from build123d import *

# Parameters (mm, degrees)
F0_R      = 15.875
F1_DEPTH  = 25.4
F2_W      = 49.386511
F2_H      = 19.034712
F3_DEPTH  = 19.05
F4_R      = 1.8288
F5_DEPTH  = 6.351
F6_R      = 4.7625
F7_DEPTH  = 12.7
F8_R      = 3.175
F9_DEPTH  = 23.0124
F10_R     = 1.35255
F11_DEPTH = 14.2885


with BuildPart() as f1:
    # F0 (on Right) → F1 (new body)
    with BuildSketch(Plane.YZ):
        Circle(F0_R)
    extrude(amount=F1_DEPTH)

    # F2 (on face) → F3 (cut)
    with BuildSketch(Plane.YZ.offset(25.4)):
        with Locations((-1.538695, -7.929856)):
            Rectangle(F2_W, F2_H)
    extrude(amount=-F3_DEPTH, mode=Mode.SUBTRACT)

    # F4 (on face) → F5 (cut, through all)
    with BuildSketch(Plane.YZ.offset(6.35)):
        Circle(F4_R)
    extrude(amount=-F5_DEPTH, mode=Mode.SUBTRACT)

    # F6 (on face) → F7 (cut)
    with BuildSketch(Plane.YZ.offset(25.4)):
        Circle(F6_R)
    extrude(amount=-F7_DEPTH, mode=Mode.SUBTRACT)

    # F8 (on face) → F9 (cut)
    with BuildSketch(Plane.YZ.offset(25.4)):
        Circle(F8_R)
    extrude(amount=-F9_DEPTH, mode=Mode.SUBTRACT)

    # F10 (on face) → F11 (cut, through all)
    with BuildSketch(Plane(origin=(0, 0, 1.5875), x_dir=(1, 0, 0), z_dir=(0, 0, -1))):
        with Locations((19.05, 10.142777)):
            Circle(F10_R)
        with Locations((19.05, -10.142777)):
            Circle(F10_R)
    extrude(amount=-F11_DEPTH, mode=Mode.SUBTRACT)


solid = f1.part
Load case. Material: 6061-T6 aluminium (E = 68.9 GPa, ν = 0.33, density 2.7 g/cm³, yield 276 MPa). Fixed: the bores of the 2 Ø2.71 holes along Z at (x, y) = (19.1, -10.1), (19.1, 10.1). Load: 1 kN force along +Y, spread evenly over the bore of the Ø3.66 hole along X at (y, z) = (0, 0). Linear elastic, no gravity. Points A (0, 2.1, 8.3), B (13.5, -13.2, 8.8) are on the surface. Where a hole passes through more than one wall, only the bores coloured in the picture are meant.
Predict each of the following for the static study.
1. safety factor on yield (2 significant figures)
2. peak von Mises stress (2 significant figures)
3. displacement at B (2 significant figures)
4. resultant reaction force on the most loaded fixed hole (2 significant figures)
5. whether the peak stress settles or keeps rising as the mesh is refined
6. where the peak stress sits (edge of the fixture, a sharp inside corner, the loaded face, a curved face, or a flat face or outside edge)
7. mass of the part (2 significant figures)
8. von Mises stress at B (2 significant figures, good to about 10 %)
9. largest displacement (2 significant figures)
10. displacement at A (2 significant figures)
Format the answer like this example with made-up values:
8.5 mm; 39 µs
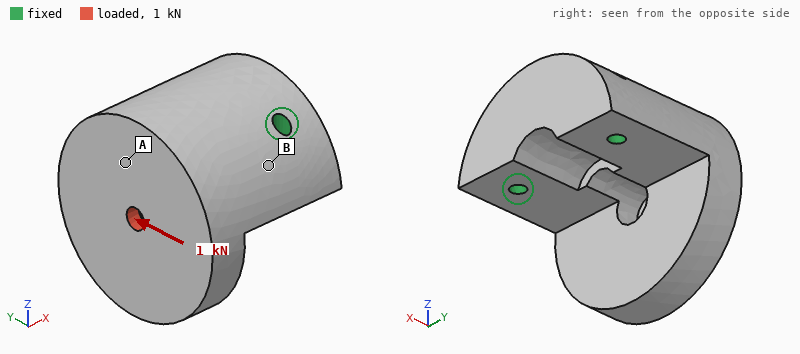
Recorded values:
4.1; 67 MPa; 2.5 µm; 1.0 kN; settles; the loaded face; 30 g; 15 MPa; 13 µm; 4.0 µm
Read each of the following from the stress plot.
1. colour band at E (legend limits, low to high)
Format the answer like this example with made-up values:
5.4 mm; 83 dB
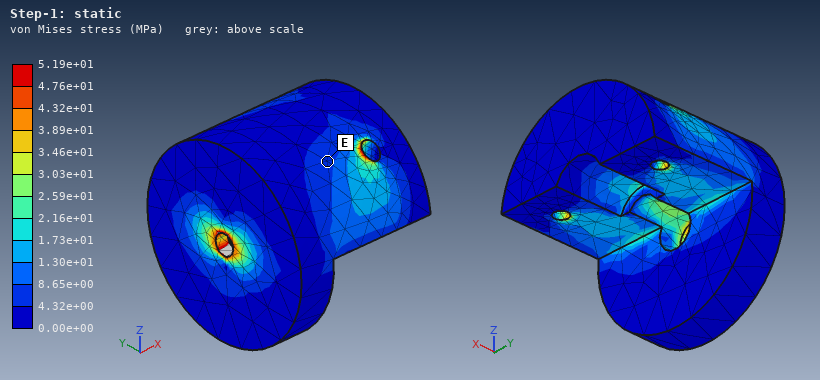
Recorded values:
4.32e+00 to 8.65e+00 MPa
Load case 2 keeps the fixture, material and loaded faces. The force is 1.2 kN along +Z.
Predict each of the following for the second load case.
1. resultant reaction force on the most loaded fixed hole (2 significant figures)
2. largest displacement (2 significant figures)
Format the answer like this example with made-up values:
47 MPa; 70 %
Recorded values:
620 N; 38 µm
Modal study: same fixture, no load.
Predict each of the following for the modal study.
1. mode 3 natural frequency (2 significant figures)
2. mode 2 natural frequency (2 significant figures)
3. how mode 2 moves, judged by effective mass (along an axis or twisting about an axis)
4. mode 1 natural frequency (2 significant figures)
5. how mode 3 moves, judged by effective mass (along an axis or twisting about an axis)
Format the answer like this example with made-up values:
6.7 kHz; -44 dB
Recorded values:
17 kHz; 13 kHz; along Y; 8800 Hz; along Z
